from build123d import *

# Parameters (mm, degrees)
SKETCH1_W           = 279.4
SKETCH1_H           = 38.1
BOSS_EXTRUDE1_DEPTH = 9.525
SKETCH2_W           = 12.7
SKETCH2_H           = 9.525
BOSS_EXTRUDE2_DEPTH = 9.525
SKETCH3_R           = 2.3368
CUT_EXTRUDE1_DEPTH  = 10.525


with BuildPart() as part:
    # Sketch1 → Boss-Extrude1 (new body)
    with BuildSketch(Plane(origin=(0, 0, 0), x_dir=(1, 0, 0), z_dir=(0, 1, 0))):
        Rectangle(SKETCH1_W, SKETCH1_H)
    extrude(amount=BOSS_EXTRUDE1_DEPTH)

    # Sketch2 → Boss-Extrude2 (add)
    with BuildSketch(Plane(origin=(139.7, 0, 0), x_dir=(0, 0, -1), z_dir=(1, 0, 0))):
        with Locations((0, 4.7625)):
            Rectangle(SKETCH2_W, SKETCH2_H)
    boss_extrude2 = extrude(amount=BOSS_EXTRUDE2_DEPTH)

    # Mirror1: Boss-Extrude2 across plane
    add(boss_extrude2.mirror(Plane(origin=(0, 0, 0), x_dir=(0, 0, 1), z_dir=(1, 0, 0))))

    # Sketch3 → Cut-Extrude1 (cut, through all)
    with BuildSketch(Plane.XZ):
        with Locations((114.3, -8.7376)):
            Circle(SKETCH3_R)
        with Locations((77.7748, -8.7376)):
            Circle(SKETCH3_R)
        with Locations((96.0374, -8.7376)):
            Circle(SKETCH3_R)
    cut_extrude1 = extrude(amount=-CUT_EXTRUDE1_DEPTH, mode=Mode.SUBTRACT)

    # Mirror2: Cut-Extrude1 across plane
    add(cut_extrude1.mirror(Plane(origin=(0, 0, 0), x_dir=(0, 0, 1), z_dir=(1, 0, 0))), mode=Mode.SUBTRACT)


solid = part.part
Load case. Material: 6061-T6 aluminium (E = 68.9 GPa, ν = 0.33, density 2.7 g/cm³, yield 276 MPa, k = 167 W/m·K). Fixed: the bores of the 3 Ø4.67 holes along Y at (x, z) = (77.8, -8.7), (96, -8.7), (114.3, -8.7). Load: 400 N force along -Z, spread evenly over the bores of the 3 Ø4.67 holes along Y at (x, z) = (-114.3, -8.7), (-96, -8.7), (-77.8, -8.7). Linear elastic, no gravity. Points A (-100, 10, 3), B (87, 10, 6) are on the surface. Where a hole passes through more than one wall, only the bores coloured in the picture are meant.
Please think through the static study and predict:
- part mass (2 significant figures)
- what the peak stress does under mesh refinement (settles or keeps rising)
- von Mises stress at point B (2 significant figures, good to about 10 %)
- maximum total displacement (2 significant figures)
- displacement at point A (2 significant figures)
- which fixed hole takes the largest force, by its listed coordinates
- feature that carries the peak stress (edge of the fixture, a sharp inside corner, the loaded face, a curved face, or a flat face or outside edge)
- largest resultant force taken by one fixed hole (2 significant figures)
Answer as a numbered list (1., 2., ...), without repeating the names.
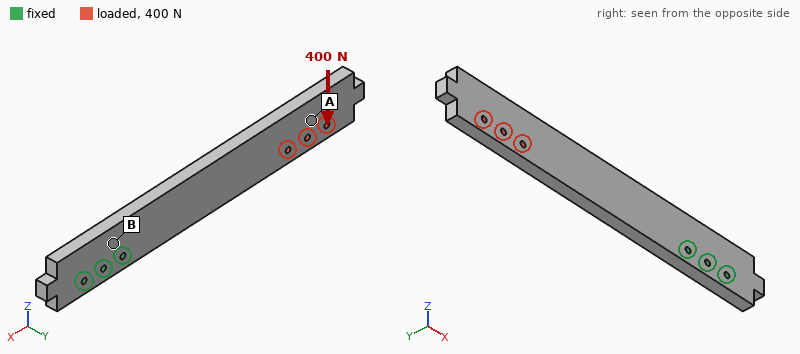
1. 280 g
2. keeps rising
3. 15 MPa
4. 0.45 mm
5. 0.32 mm
6. (77.8, -8.7)
7. edge of the fixture
8. 2.7 kN
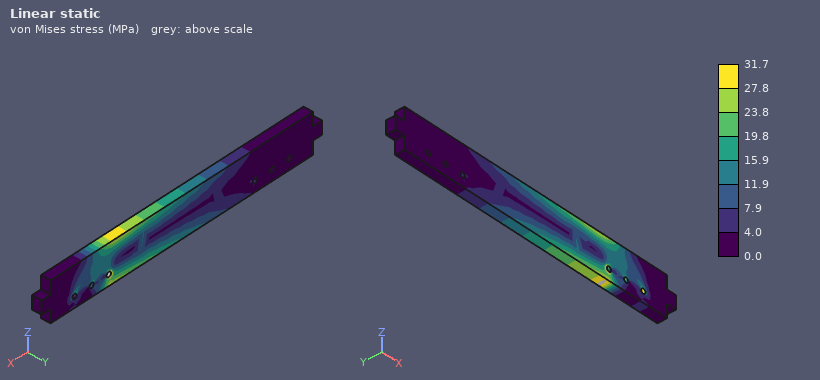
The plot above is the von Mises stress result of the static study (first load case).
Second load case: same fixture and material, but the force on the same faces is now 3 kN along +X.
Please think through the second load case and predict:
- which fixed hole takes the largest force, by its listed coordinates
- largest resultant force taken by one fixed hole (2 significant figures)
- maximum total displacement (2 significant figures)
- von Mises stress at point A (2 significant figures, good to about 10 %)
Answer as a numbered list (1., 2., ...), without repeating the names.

1. (77.8, -8.7)
2. 2.4 kN
3. 0.21 mm
4. 3.3 MPa
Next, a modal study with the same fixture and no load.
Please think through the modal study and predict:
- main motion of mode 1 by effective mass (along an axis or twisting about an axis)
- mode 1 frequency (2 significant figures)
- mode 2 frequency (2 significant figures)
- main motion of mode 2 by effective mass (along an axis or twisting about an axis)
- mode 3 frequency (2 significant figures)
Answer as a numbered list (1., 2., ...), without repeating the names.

1. along Y
2. 160 Hz
3. 540 Hz
4. along Z
5. 960 Hz
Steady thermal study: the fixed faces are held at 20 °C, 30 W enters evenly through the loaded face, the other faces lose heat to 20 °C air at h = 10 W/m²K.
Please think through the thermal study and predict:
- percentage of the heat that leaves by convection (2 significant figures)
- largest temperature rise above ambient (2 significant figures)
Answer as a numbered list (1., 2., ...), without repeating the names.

1. 30 %
2. 70 K
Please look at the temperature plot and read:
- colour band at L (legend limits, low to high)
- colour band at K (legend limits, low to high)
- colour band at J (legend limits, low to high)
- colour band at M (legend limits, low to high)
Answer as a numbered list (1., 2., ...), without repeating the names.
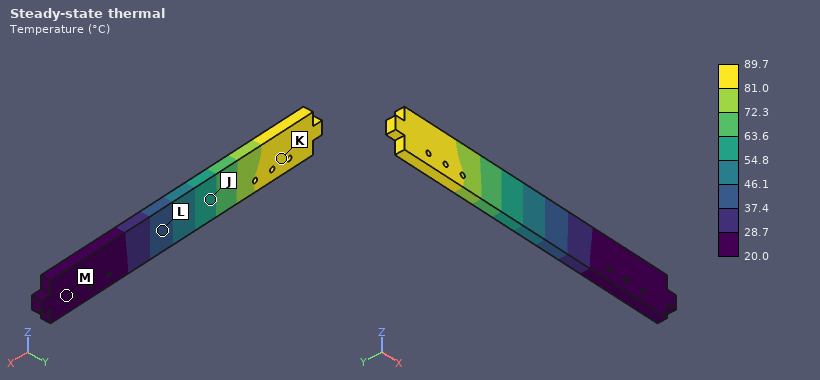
1. 37.4 to 46.1 °C
2. 81.0 to 89.7 °C
3. 54.8 to 63.6 °C
4. 20.0 to 28.7 °C
